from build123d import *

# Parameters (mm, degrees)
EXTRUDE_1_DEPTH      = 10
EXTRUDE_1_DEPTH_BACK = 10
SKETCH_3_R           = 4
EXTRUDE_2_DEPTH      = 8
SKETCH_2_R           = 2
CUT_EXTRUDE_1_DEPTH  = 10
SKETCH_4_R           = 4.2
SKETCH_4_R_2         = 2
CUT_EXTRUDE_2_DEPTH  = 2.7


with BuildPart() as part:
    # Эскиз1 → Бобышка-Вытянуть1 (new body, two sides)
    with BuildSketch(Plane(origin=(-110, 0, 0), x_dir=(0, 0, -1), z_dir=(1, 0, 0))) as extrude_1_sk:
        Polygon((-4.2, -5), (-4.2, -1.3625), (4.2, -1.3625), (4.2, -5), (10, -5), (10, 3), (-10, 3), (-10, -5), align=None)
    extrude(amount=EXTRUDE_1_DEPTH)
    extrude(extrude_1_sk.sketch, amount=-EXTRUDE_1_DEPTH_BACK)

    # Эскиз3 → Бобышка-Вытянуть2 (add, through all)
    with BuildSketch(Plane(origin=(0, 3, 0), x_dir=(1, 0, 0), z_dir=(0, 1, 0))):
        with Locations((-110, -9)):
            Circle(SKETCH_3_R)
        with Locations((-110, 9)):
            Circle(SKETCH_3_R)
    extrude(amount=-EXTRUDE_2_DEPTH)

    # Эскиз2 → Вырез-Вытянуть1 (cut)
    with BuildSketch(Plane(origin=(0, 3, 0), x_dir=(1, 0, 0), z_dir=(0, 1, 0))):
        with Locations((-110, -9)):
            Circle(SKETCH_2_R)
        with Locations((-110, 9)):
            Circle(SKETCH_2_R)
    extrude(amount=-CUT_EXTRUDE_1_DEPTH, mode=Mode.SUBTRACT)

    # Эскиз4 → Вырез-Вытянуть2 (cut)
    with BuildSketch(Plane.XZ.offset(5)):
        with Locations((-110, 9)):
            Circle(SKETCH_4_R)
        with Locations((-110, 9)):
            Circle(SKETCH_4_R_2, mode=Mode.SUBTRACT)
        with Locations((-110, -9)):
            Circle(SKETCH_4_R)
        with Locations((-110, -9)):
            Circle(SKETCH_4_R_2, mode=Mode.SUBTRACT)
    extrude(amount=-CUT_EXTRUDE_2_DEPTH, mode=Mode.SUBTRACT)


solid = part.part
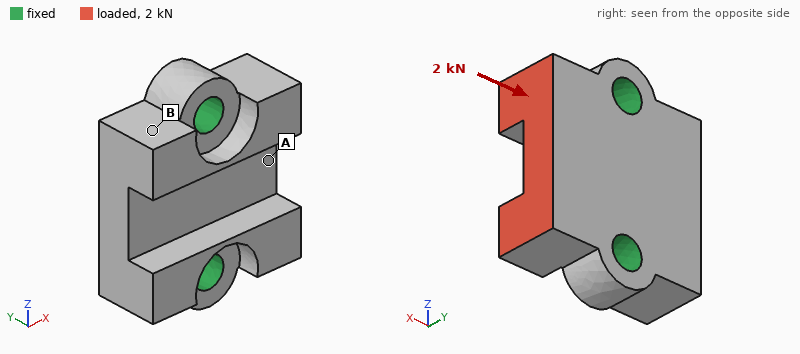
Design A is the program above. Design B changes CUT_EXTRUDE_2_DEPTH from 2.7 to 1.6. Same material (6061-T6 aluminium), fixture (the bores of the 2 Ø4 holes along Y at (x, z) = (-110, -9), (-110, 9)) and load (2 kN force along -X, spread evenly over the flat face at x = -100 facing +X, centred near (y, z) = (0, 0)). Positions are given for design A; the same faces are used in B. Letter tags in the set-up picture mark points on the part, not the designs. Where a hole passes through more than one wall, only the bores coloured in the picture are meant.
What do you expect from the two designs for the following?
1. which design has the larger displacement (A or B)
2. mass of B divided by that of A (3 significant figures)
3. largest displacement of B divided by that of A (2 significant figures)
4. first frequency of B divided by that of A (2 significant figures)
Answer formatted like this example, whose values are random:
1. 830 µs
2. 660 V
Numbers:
1. A
2. 1.04
3. 0.55
4. 1.2
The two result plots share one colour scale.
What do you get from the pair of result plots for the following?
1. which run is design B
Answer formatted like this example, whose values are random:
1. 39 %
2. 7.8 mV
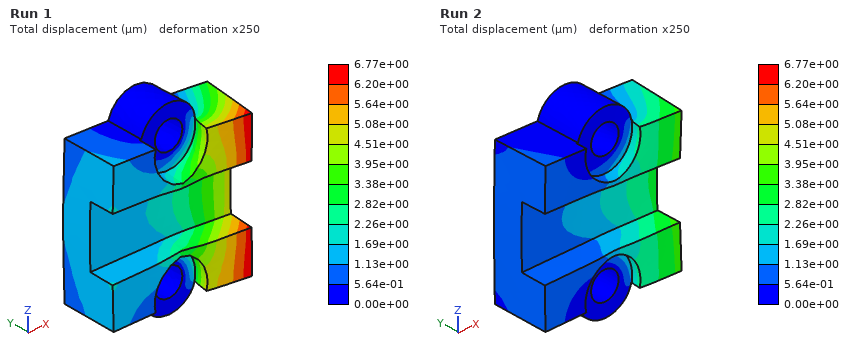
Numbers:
1. Run 2
